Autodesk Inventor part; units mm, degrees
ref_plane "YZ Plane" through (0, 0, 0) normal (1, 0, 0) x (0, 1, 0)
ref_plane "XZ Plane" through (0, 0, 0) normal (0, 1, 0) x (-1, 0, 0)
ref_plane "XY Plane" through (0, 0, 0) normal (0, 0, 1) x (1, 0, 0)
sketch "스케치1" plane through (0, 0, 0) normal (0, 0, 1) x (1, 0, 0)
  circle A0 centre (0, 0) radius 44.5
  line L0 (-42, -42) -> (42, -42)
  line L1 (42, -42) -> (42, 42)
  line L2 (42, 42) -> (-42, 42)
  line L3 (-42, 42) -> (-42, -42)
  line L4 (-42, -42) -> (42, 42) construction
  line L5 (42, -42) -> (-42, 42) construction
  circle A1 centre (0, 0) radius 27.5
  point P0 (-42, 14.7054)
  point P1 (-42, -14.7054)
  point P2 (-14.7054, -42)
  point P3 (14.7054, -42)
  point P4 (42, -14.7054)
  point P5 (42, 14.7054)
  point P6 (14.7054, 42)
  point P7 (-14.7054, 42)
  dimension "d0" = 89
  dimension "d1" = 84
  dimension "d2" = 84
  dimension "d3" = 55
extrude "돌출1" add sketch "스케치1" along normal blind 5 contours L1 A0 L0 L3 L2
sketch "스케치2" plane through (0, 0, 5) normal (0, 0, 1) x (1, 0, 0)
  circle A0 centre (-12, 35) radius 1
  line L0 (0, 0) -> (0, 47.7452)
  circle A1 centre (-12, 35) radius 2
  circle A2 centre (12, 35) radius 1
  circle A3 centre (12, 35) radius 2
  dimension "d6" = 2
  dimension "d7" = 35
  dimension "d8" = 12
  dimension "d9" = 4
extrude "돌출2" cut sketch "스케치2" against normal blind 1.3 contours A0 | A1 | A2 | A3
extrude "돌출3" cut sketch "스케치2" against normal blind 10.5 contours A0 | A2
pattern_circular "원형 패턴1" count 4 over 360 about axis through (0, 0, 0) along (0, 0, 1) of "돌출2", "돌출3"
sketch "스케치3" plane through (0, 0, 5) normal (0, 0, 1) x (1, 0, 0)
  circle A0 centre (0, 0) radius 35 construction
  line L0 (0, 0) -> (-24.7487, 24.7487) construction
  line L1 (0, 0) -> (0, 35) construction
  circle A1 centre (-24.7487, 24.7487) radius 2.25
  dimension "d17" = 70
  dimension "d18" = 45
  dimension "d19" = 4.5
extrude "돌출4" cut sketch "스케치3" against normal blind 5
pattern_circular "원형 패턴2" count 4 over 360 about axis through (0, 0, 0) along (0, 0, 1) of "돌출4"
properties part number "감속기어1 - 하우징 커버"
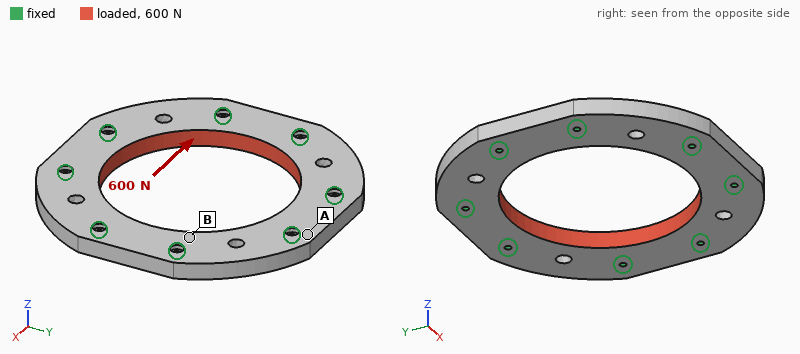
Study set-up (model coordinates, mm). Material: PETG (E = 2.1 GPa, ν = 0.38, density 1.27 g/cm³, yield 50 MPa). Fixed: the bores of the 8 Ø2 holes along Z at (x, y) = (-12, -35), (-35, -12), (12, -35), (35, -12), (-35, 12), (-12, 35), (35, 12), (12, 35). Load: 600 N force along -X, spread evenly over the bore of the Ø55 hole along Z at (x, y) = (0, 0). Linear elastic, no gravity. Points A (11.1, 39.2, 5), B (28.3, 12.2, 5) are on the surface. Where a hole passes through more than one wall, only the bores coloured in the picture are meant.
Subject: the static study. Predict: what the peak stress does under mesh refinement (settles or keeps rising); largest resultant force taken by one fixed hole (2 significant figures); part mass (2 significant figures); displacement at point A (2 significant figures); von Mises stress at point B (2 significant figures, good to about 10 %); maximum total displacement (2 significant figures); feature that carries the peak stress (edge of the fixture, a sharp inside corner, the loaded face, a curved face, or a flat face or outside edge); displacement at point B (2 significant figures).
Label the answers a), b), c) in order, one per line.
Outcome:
a) keeps rising
b) 82 N
c) 22 g
d) 2.9 µm
e) 1.2 MPa
f) 16 µm
g) edge of the fixture
h) 9.6 µm
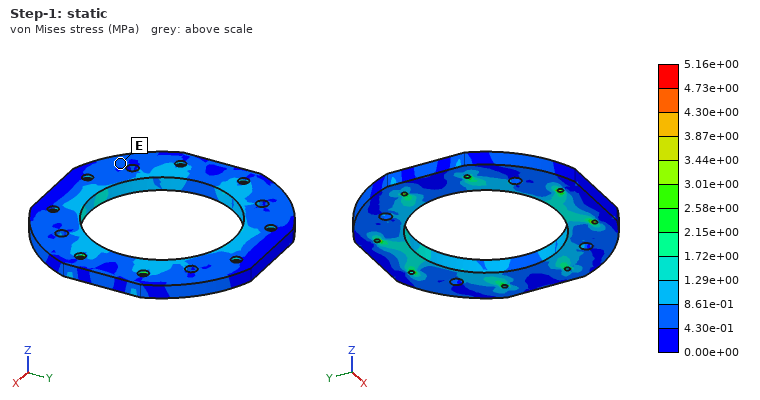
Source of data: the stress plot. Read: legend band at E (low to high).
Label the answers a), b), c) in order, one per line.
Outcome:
a) 4.30e-01 to 8.61e-01 MPa
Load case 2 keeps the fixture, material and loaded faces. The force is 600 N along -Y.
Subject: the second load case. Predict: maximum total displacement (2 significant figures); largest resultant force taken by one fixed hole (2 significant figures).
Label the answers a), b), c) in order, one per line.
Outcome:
a) 16 µm
b) 82 N
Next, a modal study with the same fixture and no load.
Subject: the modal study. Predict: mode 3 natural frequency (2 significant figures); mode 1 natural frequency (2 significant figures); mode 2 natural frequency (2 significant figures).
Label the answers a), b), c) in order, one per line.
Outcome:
a) 3700 Hz
b) 3600 Hz
c) 3700 Hz
